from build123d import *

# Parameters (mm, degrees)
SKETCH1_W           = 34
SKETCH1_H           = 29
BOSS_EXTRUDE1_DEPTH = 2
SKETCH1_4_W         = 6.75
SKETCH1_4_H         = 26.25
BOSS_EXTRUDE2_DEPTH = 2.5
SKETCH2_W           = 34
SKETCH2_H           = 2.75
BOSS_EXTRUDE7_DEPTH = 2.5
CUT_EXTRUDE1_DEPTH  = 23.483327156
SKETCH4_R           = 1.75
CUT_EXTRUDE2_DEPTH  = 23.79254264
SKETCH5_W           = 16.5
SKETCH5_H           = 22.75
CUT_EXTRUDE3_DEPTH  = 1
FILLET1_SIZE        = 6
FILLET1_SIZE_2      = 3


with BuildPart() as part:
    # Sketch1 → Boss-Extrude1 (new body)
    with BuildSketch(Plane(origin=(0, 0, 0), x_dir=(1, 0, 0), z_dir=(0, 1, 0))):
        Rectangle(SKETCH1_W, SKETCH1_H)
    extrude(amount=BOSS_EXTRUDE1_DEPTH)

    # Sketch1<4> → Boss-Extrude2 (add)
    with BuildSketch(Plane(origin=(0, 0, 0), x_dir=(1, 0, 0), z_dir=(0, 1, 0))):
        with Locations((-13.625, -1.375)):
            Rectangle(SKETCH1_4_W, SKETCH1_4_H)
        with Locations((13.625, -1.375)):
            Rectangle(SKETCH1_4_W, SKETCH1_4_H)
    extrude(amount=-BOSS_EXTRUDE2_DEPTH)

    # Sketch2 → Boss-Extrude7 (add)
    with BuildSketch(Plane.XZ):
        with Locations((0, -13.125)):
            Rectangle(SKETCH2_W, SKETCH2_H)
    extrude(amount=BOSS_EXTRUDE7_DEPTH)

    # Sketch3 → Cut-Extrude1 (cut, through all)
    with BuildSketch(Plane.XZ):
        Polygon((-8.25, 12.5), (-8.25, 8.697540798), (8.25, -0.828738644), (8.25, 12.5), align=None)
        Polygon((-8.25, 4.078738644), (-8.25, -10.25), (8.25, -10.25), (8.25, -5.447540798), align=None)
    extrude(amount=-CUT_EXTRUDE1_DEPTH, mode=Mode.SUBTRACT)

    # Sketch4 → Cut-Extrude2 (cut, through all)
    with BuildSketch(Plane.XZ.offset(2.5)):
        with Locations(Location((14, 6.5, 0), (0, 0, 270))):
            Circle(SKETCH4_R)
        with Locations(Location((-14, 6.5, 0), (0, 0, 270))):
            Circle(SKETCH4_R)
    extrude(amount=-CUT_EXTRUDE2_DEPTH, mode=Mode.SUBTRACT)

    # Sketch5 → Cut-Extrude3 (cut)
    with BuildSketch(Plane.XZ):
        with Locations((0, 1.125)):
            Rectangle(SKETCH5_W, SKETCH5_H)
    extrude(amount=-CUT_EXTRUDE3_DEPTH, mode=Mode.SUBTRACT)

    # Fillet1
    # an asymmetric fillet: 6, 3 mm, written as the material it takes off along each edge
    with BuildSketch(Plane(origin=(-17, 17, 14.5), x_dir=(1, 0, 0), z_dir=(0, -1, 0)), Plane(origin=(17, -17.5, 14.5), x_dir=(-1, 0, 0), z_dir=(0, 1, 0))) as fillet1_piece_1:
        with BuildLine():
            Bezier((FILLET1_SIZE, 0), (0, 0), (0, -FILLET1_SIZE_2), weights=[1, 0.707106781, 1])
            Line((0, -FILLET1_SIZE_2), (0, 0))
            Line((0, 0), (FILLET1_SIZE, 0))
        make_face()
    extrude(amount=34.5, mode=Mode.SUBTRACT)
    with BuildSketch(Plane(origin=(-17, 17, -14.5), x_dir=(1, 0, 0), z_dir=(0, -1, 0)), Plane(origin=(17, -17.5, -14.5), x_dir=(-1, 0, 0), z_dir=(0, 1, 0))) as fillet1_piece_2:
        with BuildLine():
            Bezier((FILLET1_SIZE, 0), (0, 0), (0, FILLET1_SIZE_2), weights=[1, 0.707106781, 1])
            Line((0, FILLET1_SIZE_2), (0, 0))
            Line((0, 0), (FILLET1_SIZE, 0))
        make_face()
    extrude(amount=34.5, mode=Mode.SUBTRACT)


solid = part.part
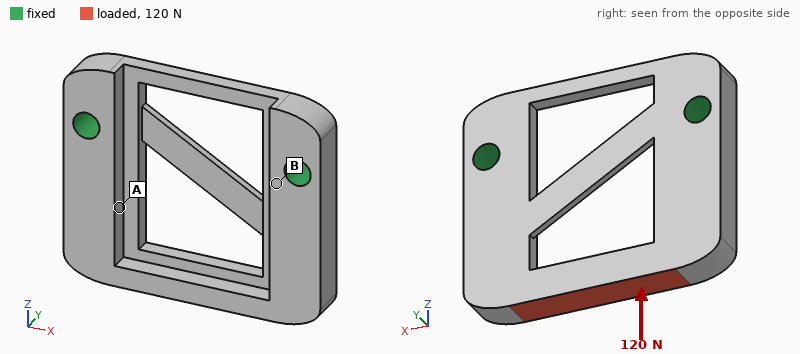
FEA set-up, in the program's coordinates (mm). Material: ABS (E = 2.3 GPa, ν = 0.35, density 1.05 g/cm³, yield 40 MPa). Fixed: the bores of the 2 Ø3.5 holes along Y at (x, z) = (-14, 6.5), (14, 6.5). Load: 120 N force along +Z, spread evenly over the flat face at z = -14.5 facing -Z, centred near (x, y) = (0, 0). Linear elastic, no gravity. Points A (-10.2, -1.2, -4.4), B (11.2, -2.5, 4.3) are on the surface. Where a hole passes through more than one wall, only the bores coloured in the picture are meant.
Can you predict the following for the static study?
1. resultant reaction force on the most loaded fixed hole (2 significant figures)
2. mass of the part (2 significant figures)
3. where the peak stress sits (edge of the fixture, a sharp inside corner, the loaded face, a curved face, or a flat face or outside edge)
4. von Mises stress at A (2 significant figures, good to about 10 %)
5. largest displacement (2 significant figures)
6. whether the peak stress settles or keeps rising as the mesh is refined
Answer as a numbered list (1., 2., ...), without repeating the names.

1. 65 N
2. 2.4 g
3. a sharp inside corner
4. 4.4 MPa
5. 0.18 mm
6. keeps rising
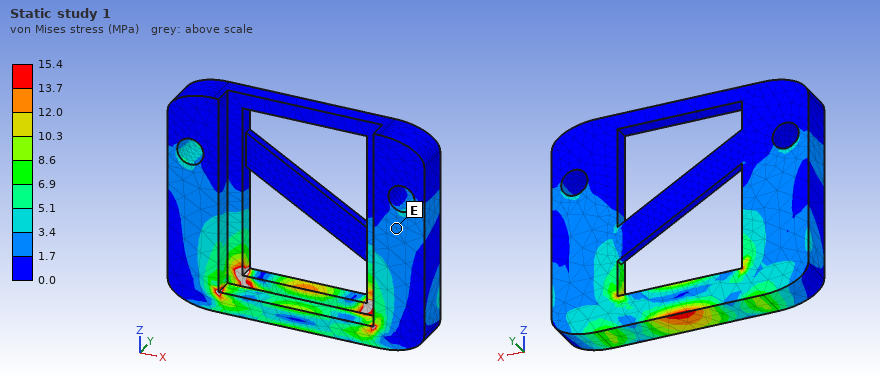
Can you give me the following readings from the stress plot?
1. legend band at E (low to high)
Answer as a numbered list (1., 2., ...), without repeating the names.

1. 1.7 to 3.4 MPa
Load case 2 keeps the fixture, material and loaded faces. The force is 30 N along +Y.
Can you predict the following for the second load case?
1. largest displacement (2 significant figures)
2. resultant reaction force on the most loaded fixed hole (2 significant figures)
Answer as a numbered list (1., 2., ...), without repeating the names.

1. 0.42 mm
2. 15 N
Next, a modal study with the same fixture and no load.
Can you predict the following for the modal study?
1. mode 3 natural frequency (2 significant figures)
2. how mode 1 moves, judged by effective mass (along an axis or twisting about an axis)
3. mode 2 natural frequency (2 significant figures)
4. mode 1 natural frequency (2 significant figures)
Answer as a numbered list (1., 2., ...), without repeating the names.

1. 3900 Hz
2. along Y
3. 3100 Hz
4. 2000 Hz
